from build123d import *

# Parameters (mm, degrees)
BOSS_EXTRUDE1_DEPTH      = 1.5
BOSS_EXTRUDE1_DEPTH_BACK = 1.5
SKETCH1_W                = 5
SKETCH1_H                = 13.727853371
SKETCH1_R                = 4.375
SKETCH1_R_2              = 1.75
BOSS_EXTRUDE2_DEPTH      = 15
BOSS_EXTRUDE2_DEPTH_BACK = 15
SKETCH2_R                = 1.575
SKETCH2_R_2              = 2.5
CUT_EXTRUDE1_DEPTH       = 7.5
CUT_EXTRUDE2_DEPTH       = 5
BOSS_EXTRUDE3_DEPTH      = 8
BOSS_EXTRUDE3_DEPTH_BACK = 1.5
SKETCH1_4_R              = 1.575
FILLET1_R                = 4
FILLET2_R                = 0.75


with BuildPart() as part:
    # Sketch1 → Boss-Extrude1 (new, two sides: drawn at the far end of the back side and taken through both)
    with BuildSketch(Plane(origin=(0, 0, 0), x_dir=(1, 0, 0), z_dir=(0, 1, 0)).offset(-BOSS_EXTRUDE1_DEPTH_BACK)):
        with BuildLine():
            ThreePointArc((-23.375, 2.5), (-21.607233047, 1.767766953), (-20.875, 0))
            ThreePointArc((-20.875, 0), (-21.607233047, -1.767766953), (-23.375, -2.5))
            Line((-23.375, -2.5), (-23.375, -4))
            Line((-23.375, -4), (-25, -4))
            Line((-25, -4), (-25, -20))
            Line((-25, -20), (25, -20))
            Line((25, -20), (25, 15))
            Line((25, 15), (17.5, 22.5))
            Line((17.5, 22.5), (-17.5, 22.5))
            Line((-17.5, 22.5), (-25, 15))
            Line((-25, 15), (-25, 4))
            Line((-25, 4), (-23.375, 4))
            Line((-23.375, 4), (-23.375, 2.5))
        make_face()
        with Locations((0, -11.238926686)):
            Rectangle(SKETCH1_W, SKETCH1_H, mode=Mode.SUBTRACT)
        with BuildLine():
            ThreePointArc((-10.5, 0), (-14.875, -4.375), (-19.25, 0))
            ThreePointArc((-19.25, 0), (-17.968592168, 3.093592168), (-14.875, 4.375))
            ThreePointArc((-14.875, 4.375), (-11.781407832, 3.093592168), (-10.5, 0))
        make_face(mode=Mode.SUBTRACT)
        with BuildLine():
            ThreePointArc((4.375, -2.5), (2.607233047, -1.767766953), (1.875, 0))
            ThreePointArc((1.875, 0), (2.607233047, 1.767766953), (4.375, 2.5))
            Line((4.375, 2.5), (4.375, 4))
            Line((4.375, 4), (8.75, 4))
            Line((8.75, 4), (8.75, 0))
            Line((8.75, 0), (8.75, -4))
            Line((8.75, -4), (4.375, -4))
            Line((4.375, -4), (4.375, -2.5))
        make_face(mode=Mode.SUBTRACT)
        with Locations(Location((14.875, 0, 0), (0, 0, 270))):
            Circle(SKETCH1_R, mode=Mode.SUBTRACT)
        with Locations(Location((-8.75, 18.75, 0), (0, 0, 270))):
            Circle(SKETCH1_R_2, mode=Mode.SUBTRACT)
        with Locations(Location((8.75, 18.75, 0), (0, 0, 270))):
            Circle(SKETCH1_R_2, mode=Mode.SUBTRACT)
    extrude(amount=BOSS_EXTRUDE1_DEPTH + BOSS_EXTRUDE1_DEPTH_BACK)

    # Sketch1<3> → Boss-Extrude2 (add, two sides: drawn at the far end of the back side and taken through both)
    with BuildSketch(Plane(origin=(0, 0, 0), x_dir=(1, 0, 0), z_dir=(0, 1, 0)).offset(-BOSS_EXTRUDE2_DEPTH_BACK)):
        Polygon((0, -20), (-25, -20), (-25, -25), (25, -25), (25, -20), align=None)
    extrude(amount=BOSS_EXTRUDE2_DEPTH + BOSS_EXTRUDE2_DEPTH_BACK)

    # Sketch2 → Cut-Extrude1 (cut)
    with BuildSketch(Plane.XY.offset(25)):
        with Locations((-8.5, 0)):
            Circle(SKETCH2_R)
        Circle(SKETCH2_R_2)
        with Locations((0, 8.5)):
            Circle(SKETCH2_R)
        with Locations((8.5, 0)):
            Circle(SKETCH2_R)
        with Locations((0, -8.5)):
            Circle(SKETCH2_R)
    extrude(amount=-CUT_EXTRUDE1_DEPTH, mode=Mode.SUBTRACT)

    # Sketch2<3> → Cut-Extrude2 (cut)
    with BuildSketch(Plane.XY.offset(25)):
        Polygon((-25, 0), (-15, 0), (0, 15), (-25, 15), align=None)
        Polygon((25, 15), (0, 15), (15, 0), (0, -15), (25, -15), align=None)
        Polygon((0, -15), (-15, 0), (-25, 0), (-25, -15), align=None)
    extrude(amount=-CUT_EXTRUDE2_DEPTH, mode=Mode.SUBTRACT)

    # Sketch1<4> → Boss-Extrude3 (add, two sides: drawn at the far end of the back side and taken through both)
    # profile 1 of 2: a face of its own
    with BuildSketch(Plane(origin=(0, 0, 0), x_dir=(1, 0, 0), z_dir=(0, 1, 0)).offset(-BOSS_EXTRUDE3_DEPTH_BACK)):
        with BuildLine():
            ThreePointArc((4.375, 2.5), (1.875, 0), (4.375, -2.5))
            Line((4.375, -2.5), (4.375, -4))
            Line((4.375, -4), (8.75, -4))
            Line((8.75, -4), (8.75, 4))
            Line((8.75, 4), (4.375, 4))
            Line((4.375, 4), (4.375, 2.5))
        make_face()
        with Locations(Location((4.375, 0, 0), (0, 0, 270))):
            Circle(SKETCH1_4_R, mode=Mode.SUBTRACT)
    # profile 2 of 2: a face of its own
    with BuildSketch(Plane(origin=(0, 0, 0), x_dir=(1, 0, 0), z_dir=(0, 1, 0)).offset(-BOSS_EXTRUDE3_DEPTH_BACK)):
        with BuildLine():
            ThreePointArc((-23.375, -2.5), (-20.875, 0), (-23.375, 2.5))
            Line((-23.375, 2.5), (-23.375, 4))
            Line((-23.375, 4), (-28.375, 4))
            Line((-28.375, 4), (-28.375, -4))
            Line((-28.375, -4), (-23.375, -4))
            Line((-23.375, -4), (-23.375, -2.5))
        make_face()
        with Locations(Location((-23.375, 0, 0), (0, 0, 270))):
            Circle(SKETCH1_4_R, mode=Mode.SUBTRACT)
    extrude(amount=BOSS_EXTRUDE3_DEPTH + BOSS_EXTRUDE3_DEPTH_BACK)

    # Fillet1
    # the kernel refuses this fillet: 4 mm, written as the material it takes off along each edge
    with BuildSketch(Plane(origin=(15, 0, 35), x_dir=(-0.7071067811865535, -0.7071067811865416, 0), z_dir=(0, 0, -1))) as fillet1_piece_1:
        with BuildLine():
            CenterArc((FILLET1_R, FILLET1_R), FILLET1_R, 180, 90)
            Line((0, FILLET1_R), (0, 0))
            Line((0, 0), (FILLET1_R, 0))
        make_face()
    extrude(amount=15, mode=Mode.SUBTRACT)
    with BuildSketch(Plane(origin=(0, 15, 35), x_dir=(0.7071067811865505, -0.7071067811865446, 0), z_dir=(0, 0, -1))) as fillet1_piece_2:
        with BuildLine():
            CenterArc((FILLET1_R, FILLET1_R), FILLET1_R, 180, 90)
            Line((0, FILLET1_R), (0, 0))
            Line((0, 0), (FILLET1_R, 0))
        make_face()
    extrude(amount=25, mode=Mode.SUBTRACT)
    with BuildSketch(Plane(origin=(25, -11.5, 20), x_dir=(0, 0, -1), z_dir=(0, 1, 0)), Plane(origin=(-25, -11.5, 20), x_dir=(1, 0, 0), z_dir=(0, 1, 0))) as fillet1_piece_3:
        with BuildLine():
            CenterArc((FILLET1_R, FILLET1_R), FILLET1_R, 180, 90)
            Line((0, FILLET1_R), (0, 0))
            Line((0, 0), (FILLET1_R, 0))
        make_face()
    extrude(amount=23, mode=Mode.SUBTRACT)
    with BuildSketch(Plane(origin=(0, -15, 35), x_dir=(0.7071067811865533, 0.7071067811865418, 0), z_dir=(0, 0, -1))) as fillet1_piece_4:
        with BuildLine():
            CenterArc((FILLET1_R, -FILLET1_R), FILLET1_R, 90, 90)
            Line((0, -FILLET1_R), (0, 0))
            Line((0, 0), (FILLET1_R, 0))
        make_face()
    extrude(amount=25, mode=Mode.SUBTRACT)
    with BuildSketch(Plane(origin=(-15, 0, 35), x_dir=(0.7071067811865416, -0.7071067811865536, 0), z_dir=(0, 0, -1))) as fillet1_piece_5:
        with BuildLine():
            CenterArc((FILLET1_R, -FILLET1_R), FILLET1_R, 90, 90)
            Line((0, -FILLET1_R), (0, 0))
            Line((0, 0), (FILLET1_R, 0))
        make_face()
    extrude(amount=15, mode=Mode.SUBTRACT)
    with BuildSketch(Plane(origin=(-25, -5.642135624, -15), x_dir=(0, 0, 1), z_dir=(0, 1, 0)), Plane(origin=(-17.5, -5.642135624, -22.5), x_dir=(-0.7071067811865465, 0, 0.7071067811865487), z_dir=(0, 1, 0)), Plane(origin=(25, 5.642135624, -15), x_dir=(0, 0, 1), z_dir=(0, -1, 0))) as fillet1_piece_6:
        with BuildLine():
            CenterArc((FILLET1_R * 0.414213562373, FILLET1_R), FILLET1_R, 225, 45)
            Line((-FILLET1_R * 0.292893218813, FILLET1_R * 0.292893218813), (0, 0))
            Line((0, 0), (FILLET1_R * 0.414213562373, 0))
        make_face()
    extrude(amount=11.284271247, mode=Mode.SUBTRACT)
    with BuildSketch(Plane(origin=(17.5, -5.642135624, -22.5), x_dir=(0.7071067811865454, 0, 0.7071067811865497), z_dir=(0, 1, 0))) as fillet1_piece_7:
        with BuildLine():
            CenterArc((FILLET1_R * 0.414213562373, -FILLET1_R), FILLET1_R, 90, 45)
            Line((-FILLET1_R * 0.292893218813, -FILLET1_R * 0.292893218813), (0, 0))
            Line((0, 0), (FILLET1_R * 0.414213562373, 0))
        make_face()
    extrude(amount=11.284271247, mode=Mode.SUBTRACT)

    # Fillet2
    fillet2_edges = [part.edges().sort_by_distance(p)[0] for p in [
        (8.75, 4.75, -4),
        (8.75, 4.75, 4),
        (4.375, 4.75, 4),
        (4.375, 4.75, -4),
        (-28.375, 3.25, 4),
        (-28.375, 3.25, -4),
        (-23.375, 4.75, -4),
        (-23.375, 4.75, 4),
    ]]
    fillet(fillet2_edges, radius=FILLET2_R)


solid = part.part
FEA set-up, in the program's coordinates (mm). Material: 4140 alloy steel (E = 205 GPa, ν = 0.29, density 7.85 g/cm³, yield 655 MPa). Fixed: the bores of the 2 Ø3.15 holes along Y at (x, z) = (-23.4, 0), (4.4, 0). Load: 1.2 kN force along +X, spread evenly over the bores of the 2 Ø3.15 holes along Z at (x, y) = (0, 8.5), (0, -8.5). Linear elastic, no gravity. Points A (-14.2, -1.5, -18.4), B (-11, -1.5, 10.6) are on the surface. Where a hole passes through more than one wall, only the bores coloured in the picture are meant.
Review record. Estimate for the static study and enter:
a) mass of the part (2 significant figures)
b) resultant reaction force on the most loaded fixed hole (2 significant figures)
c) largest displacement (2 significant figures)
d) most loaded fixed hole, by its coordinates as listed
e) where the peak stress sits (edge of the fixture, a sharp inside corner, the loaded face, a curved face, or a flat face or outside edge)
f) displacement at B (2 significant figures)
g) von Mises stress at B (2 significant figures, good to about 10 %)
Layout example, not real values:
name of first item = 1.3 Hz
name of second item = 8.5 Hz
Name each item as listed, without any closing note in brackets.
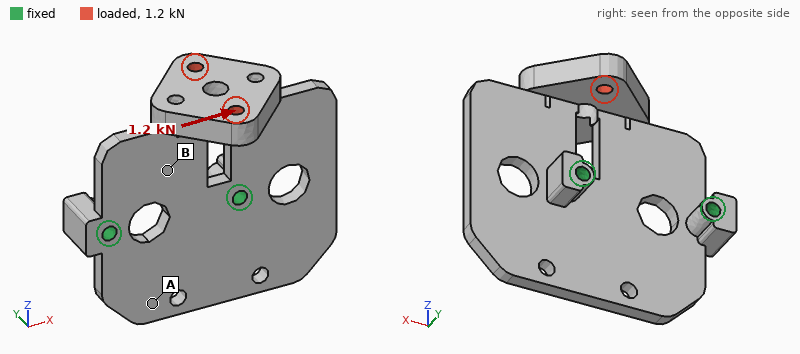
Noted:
mass of the part = 62 g
resultant reaction force on the most loaded fixed hole = 1.2 kN
largest displacement = 10 µm
most loaded fixed hole, by its coordinates as listed = (4.4, 0)
where the peak stress sits = a curved face
displacement at B = 2.9 µm
von Mises stress at B = 26 MPa
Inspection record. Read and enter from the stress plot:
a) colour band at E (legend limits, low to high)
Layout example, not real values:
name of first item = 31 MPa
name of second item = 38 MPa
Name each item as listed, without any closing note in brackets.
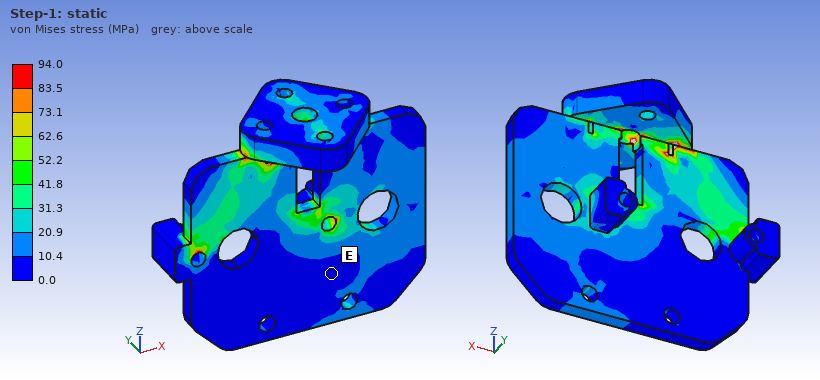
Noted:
colour band at E = 0.0 to 10.4 MPa
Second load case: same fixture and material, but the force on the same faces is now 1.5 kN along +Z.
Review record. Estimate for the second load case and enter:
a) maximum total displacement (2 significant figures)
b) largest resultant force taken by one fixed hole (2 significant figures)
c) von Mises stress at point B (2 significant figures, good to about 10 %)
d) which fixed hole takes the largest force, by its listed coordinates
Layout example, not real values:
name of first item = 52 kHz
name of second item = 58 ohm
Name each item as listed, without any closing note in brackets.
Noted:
maximum total displacement = 17 µm
largest resultant force taken by one fixed hole = 1.2 kN
von Mises stress at point B = 10 MPa
which fixed hole takes the largest force, by its listed coordinates = (4.4, 0)
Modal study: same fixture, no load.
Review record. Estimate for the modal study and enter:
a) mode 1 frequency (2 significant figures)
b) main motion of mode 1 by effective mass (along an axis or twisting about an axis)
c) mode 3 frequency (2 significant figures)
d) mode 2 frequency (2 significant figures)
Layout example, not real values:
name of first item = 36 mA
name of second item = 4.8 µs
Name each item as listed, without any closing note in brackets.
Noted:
mode 1 frequency = 2200 Hz
main motion of mode 1 by effective mass = along Y
mode 3 frequency = 4800 Hz
mode 2 frequency = 4700 Hz
